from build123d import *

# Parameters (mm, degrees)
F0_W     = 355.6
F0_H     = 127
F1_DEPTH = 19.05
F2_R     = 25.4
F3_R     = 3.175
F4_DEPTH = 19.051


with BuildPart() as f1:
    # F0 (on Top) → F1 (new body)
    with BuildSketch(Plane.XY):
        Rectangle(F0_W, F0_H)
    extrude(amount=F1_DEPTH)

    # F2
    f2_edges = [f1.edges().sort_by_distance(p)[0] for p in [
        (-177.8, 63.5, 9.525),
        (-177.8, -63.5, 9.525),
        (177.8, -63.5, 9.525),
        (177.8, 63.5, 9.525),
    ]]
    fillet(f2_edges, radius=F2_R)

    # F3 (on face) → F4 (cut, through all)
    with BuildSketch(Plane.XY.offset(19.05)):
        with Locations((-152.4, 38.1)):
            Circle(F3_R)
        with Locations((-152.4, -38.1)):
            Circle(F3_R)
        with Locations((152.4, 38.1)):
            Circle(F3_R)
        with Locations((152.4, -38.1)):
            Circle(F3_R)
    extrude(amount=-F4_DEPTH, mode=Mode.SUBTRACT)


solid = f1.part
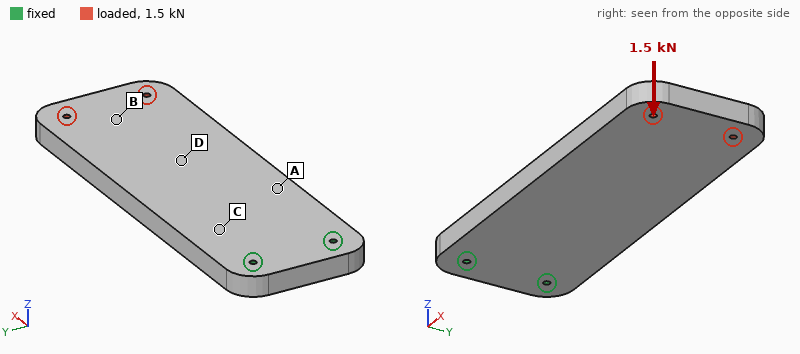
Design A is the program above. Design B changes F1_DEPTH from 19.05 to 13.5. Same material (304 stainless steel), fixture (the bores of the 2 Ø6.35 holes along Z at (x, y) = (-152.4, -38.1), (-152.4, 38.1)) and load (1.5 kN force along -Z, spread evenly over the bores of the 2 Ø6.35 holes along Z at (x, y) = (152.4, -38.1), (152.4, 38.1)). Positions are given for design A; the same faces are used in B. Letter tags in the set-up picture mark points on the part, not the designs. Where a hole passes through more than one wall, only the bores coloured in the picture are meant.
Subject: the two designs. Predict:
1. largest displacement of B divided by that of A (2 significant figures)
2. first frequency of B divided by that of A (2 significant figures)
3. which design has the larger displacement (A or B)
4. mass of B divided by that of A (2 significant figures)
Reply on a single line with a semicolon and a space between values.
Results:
2.7; 0.72; B; 0.71
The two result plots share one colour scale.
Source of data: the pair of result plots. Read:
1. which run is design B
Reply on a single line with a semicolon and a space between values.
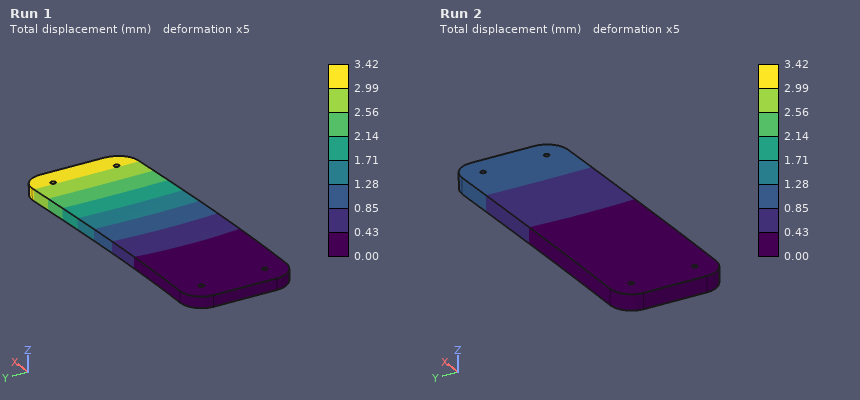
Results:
Run 1
